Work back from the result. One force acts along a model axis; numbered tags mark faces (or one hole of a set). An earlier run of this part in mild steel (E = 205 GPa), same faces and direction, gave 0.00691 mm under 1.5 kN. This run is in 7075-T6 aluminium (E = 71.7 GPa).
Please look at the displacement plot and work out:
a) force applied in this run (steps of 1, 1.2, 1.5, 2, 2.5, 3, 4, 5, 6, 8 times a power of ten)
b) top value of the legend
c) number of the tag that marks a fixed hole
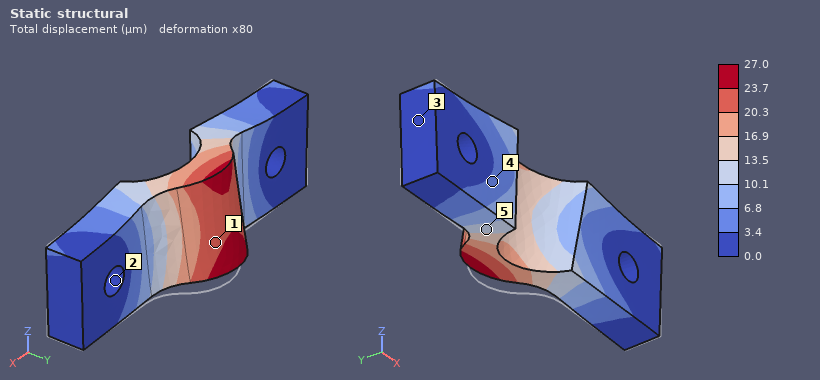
2 kN
27.0 µm
2
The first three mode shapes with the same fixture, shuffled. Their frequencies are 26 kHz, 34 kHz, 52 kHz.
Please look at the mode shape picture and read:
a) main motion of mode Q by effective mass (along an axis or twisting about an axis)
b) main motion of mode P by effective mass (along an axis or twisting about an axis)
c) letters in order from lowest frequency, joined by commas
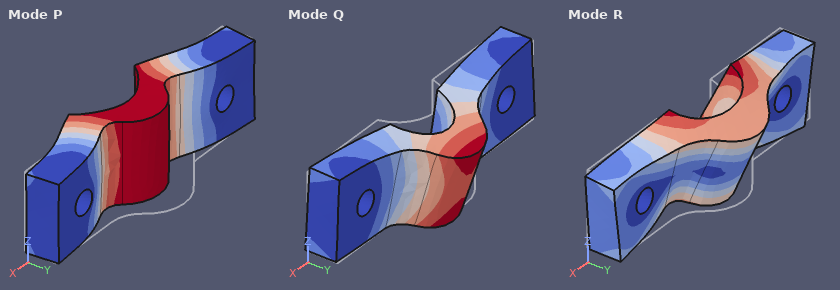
along Z
along Y
Q, P, R
